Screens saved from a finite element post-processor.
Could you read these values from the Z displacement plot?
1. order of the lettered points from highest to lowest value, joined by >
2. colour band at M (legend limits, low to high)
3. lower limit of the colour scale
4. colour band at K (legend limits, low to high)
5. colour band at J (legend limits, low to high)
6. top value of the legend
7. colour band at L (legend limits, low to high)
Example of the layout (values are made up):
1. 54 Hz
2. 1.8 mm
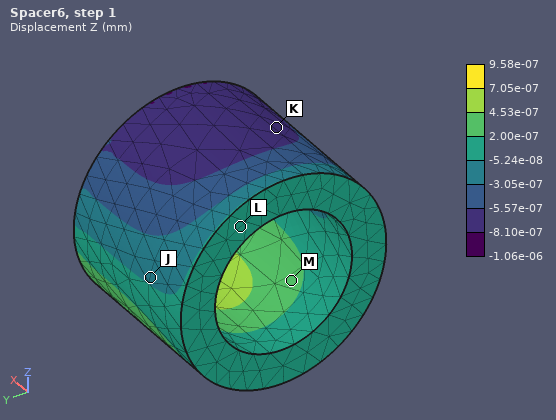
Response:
1. M > L > J > K
2. 2.00e-07 to 4.53e-07 mm
3. -1.06e-06 mm
4. -8.10e-07 to -5.57e-07 mm
5. -3.05e-07 to -5.24e-08 mm
6. 9.58e-07 mm
7. -5.24e-08 to 2.00e-07 mm
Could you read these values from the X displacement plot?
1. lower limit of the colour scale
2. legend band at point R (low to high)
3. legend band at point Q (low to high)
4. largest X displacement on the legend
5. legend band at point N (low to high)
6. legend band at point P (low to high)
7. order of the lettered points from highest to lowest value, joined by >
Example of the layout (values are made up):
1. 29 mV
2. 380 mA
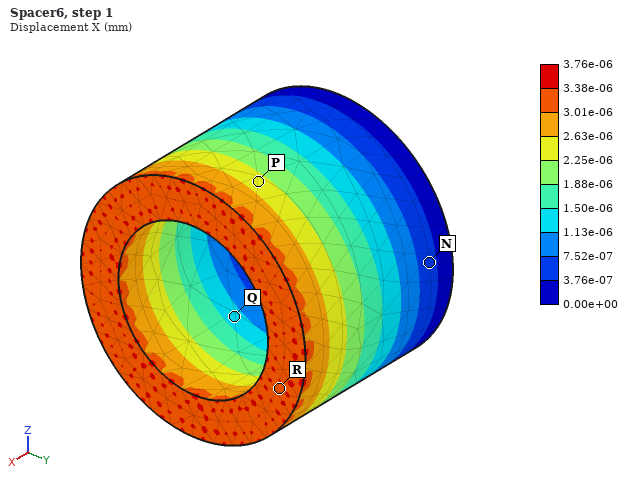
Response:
1. 0.00e+00 mm
2. 3.01e-06 to 3.38e-06 mm
3. 1.13e-06 to 1.50e-06 mm
4. 3.76e-06 mm
5. 3.76e-07 to 7.52e-07 mm
6. 2.25e-06 to 2.63e-06 mm
7. R > P > Q > N
